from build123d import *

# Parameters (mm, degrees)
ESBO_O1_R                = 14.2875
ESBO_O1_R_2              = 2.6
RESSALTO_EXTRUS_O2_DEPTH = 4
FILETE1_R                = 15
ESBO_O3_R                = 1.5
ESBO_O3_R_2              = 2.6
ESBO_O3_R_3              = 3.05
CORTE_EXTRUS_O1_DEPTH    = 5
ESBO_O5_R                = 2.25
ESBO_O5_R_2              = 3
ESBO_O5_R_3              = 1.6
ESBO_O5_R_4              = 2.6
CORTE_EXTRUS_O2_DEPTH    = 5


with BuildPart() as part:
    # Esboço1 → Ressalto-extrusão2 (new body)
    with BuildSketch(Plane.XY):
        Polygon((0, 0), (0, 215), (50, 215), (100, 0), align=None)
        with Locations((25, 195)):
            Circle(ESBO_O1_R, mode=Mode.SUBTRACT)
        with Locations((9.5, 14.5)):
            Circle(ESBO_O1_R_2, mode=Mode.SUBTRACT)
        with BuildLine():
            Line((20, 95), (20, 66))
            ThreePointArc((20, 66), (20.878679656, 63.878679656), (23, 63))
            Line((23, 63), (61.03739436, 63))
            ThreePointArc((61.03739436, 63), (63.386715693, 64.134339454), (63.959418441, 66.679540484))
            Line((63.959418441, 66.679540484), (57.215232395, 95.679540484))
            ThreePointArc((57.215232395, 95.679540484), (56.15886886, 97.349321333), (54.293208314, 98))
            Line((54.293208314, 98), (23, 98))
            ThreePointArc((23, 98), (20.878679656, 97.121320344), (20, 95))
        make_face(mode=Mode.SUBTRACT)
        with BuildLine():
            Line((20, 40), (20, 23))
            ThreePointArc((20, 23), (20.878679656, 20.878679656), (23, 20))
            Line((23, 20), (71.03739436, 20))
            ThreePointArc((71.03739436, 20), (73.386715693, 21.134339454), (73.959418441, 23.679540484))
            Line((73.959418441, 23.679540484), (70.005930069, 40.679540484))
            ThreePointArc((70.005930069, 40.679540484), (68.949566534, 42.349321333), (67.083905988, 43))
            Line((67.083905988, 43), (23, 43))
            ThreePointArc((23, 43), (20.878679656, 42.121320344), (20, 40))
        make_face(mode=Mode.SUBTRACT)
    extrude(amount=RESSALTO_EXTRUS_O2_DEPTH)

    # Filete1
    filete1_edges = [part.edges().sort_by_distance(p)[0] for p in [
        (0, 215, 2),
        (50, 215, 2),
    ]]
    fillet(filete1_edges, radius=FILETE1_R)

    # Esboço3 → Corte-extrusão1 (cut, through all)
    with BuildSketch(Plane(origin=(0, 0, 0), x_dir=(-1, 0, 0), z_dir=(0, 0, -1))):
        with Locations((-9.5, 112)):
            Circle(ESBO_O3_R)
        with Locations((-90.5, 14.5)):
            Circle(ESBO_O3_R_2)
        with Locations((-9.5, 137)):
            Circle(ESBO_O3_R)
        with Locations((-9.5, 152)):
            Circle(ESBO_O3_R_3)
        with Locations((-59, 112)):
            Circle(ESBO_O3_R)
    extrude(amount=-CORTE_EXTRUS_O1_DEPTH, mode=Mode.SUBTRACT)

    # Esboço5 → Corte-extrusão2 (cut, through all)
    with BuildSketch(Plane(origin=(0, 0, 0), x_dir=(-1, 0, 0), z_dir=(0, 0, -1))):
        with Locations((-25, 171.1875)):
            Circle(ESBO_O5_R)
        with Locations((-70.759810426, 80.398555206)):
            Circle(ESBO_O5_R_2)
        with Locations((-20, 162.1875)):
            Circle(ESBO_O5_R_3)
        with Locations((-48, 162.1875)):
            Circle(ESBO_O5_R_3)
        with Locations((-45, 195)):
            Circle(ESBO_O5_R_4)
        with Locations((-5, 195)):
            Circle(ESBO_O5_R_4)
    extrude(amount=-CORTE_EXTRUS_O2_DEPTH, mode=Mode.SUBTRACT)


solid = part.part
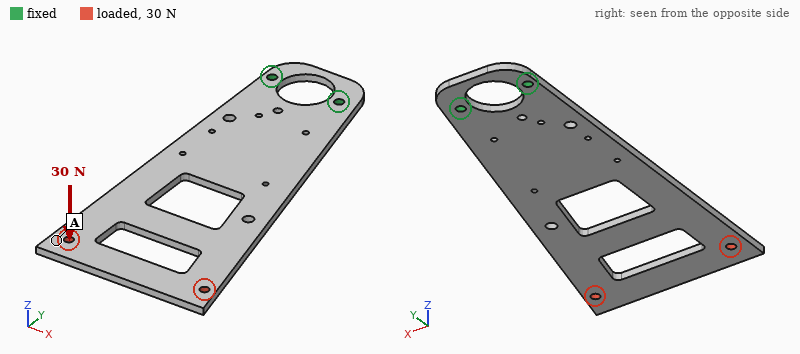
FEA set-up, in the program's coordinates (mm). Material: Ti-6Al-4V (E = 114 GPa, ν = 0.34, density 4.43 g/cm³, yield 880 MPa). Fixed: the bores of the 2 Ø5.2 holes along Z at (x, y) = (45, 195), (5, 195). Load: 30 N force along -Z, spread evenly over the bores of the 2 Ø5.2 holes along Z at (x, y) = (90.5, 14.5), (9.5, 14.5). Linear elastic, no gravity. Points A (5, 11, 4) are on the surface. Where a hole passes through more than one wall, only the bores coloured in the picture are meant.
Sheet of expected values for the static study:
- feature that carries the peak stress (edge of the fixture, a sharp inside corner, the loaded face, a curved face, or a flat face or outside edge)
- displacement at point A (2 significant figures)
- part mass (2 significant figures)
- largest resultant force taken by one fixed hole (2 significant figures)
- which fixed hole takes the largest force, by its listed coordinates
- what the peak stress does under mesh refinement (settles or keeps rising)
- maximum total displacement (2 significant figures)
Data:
edge of the fixture
2.0 mm
220 g
33 N
(45, 195)
keeps rising
2.3 mm
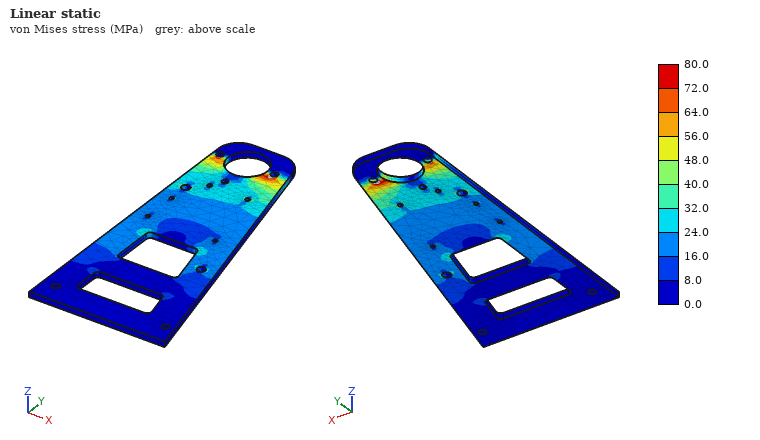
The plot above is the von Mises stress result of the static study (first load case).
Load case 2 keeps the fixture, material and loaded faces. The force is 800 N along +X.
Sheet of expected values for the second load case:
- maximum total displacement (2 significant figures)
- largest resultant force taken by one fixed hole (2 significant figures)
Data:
0.32 mm
3.4 kN
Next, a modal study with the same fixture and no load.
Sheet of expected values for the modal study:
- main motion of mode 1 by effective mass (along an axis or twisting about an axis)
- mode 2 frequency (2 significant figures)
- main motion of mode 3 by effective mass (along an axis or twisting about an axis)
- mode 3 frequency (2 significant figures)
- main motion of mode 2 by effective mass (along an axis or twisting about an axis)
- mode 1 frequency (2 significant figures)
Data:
along Z
320 Hz
along Z
430 Hz
twisting about Y
72 Hz
